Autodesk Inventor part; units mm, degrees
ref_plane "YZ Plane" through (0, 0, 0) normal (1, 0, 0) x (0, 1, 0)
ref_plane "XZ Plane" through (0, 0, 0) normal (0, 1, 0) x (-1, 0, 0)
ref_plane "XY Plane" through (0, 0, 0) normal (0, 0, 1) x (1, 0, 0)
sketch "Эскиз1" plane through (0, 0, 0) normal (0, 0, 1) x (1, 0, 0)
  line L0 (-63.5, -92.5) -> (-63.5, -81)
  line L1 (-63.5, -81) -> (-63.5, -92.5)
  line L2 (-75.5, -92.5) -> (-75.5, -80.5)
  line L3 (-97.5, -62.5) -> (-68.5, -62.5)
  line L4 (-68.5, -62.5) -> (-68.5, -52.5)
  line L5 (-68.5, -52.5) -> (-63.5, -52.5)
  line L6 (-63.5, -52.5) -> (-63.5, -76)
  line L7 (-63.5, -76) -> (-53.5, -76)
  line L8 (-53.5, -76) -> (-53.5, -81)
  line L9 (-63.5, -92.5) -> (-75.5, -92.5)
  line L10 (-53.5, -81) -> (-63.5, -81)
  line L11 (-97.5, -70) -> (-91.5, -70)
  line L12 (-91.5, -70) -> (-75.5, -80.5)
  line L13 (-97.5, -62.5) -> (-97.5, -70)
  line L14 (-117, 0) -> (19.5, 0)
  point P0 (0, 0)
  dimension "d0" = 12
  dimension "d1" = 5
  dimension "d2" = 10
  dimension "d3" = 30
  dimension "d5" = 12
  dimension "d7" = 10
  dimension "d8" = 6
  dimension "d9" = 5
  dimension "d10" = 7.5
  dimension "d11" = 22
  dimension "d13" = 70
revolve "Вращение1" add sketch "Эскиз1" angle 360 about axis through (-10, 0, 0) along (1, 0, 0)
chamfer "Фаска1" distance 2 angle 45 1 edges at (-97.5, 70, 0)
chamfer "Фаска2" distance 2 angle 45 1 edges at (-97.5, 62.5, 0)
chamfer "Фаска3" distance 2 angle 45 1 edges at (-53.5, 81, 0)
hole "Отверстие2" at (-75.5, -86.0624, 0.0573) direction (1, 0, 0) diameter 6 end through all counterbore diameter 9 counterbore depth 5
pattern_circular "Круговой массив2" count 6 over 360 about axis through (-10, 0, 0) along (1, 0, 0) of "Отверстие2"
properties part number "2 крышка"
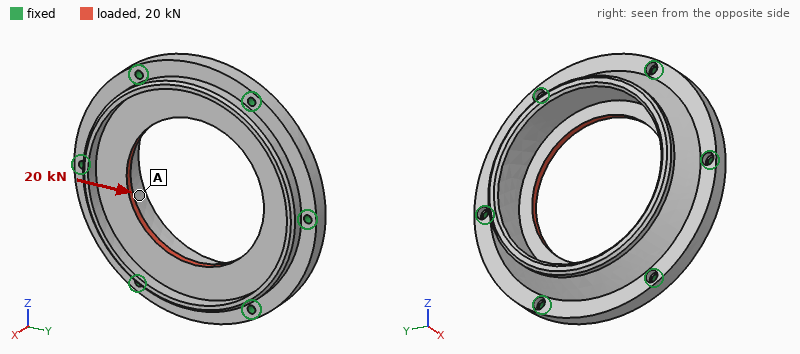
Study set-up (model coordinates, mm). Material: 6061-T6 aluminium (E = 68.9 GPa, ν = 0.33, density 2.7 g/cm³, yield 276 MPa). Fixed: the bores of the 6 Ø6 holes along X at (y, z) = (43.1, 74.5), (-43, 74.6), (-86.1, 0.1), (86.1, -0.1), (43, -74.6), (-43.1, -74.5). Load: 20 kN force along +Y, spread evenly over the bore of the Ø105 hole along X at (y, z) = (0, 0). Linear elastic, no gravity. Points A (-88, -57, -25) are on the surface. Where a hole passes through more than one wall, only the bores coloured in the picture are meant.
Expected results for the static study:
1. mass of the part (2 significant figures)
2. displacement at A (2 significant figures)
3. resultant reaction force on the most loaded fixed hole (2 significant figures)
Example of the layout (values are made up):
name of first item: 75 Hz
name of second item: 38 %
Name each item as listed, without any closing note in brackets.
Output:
mass of the part: 860 g
displacement at A: 4.3 µm
resultant reaction force on the most loaded fixed hole: 3.8 kN
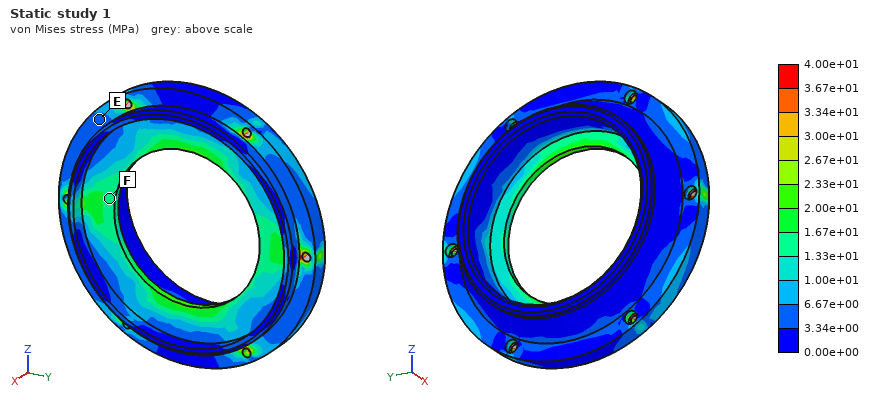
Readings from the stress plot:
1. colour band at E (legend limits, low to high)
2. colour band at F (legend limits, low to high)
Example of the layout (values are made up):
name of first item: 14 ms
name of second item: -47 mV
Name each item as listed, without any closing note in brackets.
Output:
colour band at E: 3.34e+00 to 6.67e+00 MPa
colour band at F: 1.33e+01 to 1.67e+01 MPa
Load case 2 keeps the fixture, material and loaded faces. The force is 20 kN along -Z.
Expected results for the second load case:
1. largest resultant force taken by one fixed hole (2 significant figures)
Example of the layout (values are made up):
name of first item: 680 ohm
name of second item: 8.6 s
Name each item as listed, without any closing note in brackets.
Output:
largest resultant force taken by one fixed hole: 3.6 kN
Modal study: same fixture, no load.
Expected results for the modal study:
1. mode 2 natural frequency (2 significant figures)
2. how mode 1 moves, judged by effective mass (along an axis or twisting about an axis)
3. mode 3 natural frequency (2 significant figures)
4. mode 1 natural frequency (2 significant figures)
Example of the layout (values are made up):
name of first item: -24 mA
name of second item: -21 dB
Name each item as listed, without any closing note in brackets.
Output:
mode 2 natural frequency: 7000 Hz
how mode 1 moves, judged by effective mass: along X
mode 3 natural frequency: 7000 Hz
mode 1 natural frequency: 6200 Hz
